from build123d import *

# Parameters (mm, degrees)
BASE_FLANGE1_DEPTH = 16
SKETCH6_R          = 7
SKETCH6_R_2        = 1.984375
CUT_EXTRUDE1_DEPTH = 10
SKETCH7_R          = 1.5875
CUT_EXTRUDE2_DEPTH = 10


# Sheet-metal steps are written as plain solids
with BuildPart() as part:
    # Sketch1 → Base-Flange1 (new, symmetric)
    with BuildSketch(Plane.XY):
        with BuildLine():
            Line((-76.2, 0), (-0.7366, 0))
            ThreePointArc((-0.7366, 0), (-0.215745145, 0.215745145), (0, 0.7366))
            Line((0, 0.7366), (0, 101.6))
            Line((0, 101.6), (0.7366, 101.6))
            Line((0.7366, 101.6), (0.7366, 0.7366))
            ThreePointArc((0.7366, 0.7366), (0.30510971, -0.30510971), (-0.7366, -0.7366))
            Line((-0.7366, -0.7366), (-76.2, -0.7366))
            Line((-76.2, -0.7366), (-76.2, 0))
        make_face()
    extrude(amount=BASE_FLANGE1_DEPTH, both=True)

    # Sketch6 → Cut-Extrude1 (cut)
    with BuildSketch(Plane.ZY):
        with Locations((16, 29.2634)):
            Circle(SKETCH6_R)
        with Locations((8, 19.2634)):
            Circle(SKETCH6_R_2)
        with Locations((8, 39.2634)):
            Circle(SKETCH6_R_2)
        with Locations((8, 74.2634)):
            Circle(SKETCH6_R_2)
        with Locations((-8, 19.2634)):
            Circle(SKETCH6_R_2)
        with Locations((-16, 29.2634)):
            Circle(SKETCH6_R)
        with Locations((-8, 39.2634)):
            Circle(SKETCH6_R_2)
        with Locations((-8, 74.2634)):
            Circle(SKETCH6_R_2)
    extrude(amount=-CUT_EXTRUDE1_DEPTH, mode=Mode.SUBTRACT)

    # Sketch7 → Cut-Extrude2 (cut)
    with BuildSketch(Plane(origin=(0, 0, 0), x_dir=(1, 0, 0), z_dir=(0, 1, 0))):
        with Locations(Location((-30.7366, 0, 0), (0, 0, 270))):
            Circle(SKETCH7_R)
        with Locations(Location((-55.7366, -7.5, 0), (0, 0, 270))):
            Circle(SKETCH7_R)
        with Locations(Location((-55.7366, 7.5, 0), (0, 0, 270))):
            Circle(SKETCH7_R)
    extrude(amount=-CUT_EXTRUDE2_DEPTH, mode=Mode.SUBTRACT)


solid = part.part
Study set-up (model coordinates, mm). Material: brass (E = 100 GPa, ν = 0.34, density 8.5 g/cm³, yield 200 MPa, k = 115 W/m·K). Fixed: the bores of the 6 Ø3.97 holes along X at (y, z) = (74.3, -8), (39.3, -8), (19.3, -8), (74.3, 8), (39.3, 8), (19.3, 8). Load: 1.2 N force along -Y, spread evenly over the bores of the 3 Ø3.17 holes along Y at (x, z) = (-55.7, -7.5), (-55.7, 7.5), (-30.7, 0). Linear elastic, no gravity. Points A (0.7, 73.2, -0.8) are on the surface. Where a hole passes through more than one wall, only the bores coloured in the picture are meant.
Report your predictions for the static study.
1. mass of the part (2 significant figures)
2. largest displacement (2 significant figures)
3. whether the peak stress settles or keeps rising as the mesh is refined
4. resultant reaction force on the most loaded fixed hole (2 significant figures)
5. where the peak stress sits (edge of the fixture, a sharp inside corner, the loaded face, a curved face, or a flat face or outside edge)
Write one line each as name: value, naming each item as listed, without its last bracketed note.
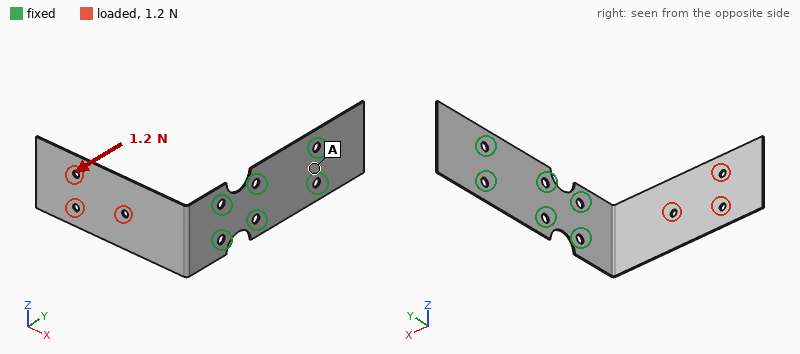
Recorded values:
mass of the part: 34 g
largest displacement: 1.5 mm
whether the peak stress settles or keeps rising as the mesh is refined: keeps rising
resultant reaction force on the most loaded fixed hole: 0.68 N
where the peak stress sits: edge of the fixture
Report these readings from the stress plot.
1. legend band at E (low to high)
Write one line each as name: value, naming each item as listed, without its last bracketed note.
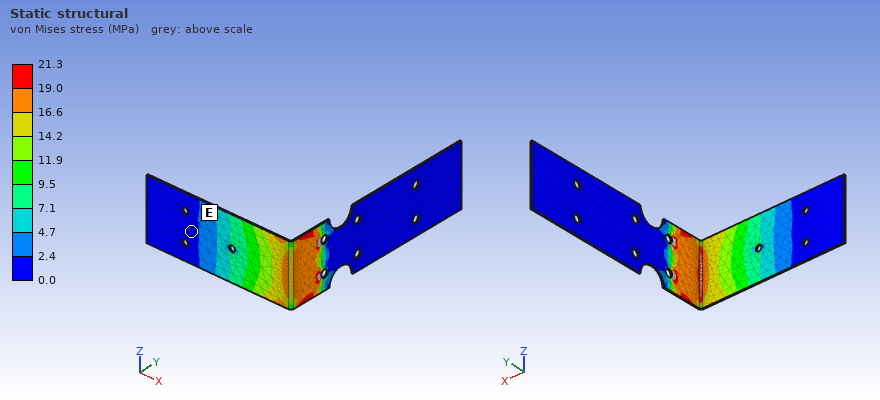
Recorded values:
legend band at E: 0.0 to 2.4 MPa
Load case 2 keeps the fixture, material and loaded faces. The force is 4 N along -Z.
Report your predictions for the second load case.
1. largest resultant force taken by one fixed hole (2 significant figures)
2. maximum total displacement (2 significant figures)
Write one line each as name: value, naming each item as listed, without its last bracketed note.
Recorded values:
largest resultant force taken by one fixed hole: 10 N
maximum total displacement: 0.84 mm
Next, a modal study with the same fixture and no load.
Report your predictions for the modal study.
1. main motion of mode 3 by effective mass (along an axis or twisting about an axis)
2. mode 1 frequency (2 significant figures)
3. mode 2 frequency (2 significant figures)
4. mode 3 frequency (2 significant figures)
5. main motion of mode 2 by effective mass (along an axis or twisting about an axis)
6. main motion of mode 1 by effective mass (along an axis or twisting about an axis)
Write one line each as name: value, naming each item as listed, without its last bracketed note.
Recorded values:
main motion of mode 3 by effective mass: along X
mode 1 frequency: 51 Hz
mode 2 frequency: 120 Hz
mode 3 frequency: 300 Hz
main motion of mode 2 by effective mass: along Z
main motion of mode 1 by effective mass: along Y
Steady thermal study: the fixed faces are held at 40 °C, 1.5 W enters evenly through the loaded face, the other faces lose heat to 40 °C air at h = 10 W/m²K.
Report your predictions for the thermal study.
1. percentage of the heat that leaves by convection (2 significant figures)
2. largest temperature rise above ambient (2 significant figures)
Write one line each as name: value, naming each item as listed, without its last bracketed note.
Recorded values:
percentage of the heat that leaves by convection: 52 %
largest temperature rise above ambient: 21 K
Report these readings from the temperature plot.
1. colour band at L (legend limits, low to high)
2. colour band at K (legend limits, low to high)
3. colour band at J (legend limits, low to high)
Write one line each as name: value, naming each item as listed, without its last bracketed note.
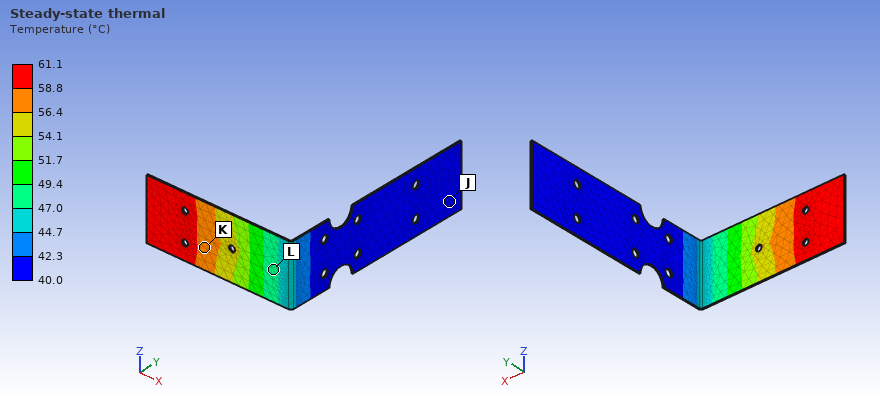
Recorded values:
colour band at L: 47.0 to 49.4 °C
colour band at K: 56.4 to 58.8 °C
colour band at J: 40.0 to 42.3 °C
